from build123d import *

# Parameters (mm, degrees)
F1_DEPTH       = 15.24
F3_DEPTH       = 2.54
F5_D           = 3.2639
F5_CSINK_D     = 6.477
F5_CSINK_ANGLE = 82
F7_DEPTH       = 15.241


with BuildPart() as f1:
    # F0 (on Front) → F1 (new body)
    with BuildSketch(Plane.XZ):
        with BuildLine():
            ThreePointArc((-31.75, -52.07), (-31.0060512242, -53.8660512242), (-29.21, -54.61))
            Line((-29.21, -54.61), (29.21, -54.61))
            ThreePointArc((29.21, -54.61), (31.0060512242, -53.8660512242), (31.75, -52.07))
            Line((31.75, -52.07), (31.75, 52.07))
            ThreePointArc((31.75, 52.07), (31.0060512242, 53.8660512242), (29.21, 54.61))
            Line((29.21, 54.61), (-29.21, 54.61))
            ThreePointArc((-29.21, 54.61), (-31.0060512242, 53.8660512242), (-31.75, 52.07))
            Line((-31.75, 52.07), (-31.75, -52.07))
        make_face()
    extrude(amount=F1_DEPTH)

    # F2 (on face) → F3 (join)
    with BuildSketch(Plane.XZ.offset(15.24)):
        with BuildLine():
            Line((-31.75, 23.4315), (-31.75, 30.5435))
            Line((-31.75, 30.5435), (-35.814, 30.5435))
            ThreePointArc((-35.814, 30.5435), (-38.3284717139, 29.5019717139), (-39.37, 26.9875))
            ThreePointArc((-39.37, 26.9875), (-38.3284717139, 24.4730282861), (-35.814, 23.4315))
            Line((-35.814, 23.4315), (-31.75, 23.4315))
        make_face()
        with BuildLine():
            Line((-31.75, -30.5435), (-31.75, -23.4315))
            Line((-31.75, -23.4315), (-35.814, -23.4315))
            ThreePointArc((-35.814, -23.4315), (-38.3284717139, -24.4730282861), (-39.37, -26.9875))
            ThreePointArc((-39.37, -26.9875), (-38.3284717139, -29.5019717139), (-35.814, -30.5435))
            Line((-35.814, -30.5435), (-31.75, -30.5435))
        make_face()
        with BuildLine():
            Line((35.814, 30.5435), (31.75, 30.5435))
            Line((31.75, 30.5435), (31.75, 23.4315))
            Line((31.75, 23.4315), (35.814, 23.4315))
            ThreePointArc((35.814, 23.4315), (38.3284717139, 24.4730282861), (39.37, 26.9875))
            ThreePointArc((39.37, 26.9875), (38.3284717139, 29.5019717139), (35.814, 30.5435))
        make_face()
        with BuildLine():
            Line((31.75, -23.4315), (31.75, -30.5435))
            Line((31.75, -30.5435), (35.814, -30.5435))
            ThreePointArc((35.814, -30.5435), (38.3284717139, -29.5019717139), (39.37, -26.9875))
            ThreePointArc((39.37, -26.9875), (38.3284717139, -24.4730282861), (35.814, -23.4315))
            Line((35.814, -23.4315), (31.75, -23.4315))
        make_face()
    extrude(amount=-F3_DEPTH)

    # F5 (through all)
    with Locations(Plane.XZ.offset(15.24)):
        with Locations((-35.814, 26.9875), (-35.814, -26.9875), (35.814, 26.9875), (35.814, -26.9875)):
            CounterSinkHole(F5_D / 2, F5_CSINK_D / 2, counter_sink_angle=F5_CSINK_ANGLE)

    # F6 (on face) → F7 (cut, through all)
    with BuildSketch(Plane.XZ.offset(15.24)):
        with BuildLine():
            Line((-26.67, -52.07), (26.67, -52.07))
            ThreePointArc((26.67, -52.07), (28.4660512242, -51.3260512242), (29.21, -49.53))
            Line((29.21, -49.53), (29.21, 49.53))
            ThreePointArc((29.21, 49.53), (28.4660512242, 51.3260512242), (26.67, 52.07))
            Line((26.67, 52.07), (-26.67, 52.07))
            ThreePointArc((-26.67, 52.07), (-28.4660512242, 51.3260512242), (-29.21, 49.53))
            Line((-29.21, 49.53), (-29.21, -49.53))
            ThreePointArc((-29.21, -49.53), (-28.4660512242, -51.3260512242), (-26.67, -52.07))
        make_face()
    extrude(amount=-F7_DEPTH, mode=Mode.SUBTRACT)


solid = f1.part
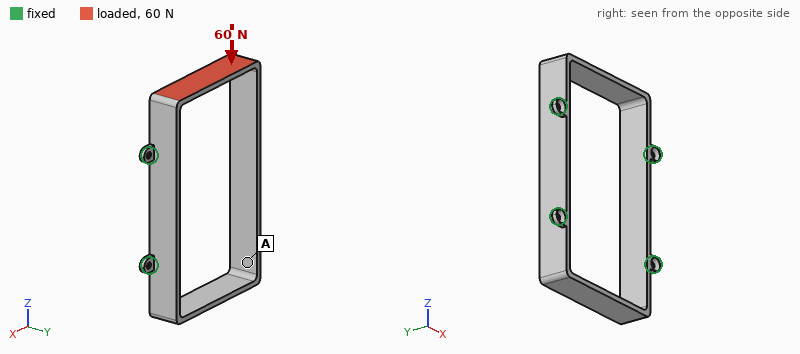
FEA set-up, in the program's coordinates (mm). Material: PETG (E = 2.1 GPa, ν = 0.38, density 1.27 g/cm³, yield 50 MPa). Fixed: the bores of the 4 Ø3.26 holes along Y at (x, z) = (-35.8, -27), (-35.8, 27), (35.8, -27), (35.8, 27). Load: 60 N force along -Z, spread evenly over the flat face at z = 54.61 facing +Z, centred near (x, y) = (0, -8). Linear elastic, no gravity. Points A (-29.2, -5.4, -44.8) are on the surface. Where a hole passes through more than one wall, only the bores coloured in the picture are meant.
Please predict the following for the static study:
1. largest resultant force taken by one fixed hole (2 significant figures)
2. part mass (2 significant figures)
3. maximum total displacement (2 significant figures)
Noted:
27 N
17 g
1.3 mm
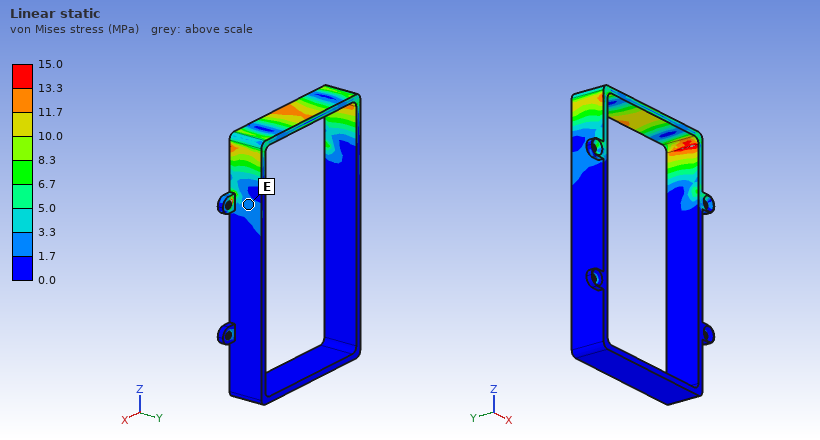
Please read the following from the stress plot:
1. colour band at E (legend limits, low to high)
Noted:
1.7 to 3.3 MPa
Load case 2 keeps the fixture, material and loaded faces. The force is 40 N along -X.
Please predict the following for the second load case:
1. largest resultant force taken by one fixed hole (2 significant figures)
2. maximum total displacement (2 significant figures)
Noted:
30 N
1.4 mm
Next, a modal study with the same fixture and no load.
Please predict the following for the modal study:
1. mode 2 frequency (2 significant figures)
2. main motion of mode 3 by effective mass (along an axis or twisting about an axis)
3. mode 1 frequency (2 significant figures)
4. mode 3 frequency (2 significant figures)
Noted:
430 Hz
along Z
430 Hz
650 Hz
